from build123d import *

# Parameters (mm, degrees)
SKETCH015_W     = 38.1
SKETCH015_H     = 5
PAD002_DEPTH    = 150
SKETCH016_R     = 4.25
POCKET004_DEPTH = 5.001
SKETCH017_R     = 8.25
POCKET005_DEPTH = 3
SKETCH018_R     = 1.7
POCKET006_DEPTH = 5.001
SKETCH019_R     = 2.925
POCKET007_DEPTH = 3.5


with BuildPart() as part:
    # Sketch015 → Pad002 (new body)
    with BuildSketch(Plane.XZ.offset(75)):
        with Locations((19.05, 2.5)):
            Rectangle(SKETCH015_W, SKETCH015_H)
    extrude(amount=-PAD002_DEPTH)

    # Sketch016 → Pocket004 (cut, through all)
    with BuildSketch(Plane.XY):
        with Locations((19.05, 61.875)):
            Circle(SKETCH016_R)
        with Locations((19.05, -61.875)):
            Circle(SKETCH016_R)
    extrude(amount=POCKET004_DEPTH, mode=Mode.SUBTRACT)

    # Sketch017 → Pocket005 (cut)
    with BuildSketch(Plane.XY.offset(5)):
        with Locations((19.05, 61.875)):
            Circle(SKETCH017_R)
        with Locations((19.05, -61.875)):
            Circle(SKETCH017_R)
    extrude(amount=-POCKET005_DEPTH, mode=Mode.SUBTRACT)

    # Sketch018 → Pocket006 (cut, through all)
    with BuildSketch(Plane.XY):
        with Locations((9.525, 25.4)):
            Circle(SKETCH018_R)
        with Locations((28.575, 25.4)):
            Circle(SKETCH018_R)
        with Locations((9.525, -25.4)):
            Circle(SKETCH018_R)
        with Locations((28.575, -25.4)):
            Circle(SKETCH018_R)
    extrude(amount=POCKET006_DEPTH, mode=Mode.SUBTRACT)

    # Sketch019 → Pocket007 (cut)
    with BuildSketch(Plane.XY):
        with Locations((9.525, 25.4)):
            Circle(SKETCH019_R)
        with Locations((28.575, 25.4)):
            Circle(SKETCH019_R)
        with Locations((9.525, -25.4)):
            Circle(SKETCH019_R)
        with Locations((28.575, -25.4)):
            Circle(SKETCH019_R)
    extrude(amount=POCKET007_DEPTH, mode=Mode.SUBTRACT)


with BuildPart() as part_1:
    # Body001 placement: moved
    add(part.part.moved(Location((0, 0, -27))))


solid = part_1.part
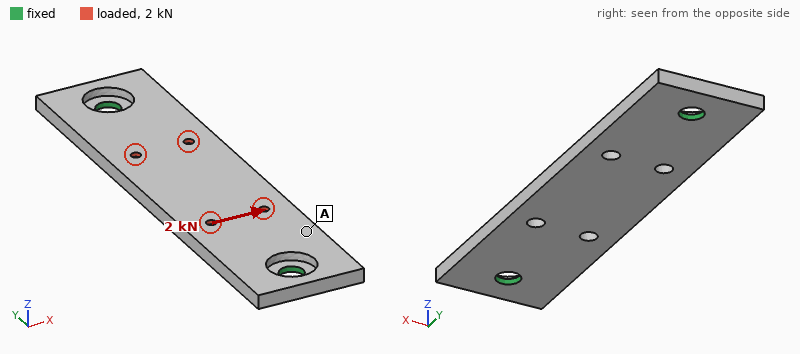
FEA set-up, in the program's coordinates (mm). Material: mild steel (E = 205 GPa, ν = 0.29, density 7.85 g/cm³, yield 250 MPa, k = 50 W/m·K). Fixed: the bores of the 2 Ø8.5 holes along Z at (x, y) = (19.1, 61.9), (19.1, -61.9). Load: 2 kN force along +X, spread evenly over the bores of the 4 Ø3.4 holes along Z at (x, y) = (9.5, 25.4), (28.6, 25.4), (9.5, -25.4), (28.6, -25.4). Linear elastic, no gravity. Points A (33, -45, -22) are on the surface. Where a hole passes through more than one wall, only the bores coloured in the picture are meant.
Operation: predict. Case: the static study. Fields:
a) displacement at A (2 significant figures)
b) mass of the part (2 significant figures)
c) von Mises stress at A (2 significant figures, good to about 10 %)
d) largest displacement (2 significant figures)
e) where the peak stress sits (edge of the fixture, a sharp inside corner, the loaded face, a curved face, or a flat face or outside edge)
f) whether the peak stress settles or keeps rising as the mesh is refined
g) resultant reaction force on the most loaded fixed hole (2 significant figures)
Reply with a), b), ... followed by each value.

a) 16 µm
b) 210 g
c) 13 MPa
d) 28 µm
e) edge of the fixture
f) keeps rising
g) 1.0 kN
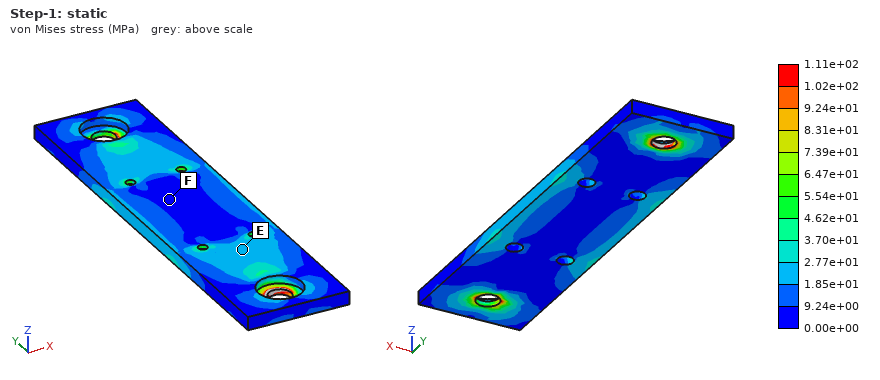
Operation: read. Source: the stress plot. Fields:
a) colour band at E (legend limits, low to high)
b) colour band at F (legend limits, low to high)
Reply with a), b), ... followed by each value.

a) 1.85e+01 to 2.77e+01 MPa
b) 0.00e+00 to 9.24e+00 MPa
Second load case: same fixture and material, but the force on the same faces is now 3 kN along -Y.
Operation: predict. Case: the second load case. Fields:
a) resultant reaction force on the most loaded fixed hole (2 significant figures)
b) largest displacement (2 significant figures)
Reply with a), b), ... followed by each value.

a) 1.5 kN
b) 4.5 µm
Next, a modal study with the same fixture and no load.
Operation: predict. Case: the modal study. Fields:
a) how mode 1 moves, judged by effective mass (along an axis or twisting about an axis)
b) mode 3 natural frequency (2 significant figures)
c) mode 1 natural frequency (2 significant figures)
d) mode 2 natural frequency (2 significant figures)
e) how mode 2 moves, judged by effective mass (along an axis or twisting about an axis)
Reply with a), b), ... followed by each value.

a) along Z
b) 3700 Hz
c) 1400 Hz
d) 2500 Hz
e) twisting about Y
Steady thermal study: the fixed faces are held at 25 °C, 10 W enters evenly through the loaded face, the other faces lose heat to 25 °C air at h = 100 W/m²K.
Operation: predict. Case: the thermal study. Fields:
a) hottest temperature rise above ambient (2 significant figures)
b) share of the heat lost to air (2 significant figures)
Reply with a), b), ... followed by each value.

a) 14 K
b) 72 %
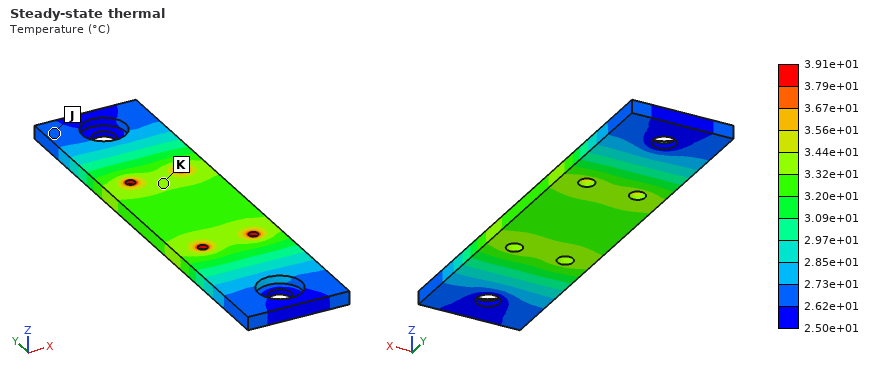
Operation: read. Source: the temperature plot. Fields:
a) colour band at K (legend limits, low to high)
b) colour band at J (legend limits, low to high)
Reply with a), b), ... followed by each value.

a) 3.32e+01 to 3.44e+01 °C
b) 2.62e+01 to 2.73e+01 °C
